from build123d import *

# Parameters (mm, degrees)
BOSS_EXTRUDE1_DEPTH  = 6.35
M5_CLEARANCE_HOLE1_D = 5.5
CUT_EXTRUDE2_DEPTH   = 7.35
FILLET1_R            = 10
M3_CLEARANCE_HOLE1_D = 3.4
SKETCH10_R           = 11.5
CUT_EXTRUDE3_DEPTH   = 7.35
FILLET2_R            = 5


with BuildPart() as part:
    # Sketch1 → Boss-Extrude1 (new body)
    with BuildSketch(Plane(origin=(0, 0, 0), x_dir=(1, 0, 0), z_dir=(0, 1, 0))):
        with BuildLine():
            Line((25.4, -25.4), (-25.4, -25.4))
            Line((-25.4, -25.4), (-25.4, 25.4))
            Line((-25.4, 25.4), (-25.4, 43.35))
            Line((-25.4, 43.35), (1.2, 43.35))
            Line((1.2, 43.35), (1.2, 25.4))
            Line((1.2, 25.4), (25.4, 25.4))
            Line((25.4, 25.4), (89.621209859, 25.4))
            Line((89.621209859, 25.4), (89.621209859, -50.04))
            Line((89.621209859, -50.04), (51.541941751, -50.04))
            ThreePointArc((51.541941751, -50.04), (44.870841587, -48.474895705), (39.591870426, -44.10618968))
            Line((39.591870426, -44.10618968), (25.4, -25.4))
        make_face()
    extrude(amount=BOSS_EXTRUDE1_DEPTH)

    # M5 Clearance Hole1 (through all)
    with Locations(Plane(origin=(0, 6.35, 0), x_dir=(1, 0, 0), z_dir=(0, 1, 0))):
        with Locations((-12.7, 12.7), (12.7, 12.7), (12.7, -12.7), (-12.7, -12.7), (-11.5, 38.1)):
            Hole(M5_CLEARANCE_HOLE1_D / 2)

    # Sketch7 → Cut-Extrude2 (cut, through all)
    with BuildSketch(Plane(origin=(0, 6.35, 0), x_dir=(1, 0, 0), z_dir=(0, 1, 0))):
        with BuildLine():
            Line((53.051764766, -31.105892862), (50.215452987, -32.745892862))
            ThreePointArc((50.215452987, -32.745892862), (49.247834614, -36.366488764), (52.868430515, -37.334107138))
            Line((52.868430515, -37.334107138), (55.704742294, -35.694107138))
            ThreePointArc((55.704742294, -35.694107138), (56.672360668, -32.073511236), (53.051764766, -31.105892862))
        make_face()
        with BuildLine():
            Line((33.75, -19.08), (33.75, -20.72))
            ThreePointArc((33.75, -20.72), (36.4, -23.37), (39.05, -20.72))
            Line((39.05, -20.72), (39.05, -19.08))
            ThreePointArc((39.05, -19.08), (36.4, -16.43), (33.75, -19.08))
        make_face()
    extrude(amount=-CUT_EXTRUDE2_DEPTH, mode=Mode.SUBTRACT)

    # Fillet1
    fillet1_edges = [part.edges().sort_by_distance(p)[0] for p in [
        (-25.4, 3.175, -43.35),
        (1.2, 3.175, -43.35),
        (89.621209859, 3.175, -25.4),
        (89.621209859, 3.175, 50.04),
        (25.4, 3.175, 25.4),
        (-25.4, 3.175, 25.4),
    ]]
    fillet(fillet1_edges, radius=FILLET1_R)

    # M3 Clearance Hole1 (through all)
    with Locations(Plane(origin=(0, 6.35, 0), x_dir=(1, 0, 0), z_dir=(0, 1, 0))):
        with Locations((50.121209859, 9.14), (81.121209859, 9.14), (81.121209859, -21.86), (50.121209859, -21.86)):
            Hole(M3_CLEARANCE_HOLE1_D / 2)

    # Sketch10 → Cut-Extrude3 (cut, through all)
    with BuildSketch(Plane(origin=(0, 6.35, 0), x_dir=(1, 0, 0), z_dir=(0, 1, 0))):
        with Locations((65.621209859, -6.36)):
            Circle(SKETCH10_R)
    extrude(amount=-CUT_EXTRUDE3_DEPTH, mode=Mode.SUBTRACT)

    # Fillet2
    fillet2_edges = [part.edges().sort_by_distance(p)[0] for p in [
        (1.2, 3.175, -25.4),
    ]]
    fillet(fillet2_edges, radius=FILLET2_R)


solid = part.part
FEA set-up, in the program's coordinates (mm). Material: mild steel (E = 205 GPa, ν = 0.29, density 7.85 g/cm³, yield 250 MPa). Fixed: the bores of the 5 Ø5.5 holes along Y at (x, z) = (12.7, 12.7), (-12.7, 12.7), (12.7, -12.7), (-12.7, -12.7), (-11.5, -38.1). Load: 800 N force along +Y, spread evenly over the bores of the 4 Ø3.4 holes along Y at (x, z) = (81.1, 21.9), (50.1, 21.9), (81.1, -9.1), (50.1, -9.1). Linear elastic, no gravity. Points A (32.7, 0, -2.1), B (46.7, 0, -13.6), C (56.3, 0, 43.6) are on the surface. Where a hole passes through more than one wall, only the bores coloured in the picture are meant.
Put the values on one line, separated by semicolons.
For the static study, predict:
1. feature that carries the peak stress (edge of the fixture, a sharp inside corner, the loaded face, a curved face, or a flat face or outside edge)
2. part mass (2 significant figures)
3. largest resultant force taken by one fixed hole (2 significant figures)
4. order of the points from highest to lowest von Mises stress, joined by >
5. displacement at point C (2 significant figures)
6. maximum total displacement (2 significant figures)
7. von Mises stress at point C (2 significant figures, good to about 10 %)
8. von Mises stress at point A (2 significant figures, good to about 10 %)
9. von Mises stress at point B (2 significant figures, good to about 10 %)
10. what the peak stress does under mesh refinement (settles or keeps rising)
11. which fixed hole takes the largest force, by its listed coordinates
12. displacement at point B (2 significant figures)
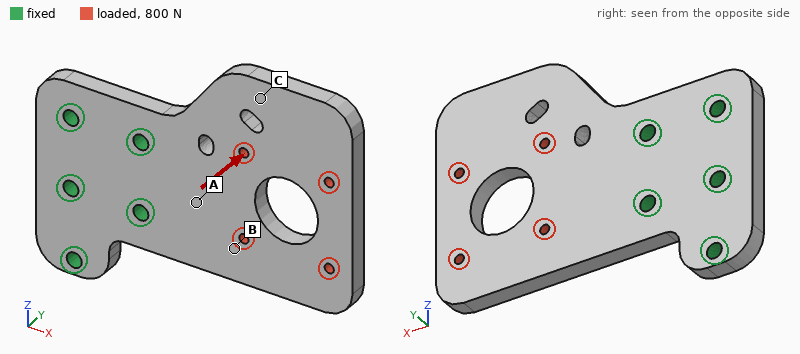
edge of the fixture; 350 g; 760 N; A > B > C; 0.14 mm; 0.31 mm; 17 MPa; 68 MPa; 46 MPa; keeps rising; (12.7, 12.7); 0.079 mm
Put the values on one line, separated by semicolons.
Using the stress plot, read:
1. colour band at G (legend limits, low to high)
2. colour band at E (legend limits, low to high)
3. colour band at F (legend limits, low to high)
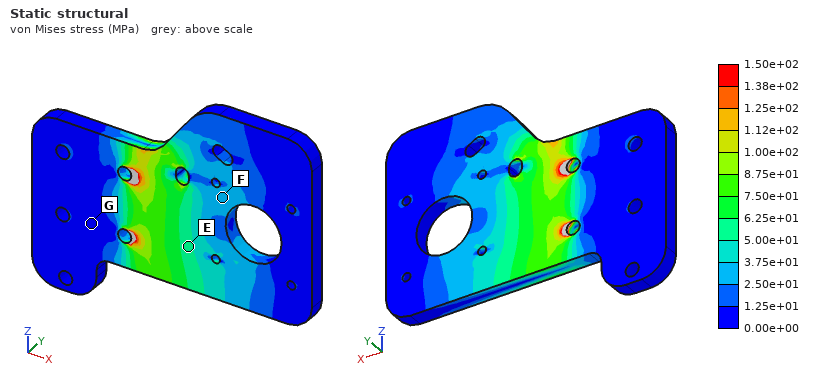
0.00e+00 to 1.25e+01 MPa; 5.00e+01 to 6.25e+01 MPa; 2.50e+01 to 3.75e+01 MPa
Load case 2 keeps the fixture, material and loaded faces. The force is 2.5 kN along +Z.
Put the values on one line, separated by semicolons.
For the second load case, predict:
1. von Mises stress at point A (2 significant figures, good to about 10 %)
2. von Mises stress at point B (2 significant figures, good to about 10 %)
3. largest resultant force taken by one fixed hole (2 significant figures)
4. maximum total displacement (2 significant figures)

26 MPa; 13 MPa; 3.6 kN; 31 µm
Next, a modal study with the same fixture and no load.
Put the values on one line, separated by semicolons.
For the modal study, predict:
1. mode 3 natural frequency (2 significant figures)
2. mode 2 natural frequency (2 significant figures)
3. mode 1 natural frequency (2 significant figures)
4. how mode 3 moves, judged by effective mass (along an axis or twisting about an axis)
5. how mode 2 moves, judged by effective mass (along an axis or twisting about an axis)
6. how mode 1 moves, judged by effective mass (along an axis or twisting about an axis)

4000 Hz; 1700 Hz; 770 Hz; along Z; twisting about X; along Y
